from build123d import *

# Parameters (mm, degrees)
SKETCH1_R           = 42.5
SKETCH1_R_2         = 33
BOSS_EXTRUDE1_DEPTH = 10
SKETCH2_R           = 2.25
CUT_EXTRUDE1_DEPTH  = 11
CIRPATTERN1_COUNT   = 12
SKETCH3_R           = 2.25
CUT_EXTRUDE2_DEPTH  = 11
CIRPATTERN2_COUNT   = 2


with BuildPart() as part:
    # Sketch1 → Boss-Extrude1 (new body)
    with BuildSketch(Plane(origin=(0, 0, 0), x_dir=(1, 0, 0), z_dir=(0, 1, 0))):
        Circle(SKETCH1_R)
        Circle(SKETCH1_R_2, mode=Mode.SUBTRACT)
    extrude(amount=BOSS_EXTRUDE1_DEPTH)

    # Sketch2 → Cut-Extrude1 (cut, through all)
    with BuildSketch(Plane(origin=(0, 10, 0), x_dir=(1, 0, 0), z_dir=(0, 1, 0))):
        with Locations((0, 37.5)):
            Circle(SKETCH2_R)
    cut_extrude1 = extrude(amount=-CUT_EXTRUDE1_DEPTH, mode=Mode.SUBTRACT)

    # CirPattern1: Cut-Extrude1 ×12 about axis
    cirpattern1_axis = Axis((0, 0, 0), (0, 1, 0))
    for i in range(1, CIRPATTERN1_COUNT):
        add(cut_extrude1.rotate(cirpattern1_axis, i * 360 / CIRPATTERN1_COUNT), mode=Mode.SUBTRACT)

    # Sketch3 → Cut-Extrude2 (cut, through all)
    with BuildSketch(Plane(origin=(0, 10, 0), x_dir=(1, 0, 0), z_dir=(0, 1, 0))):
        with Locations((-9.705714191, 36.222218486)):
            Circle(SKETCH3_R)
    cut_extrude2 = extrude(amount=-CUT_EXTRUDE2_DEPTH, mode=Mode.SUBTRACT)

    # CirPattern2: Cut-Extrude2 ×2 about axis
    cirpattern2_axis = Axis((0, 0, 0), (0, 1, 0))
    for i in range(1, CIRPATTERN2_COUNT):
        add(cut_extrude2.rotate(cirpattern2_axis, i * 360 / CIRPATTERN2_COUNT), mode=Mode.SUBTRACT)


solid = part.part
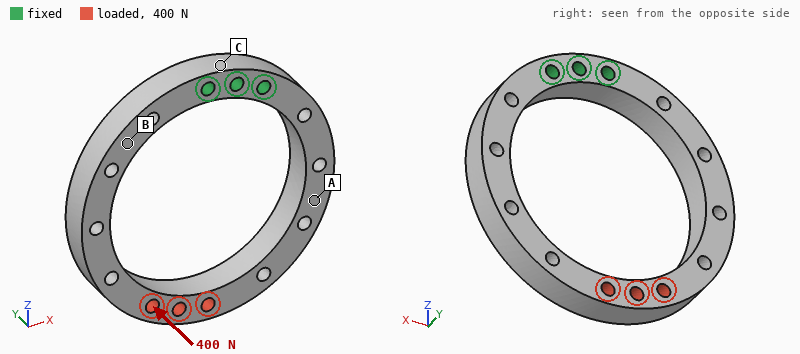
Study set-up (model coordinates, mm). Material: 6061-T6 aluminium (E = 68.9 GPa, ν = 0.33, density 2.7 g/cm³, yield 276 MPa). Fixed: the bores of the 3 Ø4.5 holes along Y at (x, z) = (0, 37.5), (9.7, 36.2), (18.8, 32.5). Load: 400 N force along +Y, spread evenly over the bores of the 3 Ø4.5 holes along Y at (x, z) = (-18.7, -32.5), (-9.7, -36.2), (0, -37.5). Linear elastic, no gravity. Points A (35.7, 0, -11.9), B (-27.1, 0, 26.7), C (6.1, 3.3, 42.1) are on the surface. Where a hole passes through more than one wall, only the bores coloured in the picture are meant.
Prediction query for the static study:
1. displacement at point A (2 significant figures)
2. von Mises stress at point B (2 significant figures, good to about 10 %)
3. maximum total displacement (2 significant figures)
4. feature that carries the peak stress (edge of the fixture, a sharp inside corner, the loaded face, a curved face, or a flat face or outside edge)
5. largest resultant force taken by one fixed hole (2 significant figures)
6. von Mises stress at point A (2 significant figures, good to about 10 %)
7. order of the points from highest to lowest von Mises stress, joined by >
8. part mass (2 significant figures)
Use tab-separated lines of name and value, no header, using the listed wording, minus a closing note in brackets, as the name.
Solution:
displacement at point A	0.40 mm
von Mises stress at point B	77 MPa
maximum total displacement	1.2 mm
feature that carries the peak stress	a curved face
largest resultant force taken by one fixed hole	240 N
von Mises stress at point A	40 MPa
order of the points from highest to lowest von Mises stress, joined by >	B > A > C
part mass	55 g
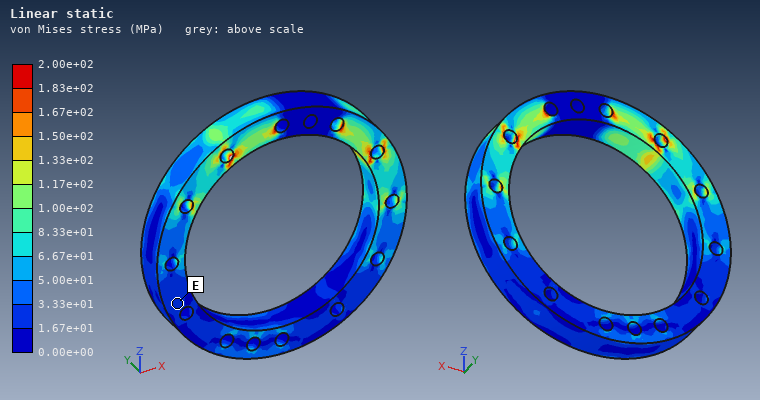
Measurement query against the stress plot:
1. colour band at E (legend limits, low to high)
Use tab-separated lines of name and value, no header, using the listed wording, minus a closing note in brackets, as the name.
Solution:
colour band at E	1.67e+01 to 3.33e+01 MPa
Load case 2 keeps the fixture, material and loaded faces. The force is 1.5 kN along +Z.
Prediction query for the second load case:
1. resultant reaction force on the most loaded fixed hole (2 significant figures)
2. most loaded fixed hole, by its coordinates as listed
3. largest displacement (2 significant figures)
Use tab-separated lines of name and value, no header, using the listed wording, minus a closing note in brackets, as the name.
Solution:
resultant reaction force on the most loaded fixed hole	1.6 kN
most loaded fixed hole, by its coordinates as listed	(0, 37.5)
largest displacement	0.37 mm
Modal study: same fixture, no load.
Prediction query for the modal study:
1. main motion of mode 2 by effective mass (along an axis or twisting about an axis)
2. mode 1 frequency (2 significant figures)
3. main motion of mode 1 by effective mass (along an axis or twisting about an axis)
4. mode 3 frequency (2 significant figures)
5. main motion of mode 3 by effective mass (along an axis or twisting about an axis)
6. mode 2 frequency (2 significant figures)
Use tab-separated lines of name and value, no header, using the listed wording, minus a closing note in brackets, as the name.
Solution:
main motion of mode 2 by effective mass	along X
mode 1 frequency	730 Hz
main motion of mode 1 by effective mass	along Y
mode 3 frequency	1800 Hz
main motion of mode 3 by effective mass	twisting about Z
mode 2 frequency	1100 Hz
